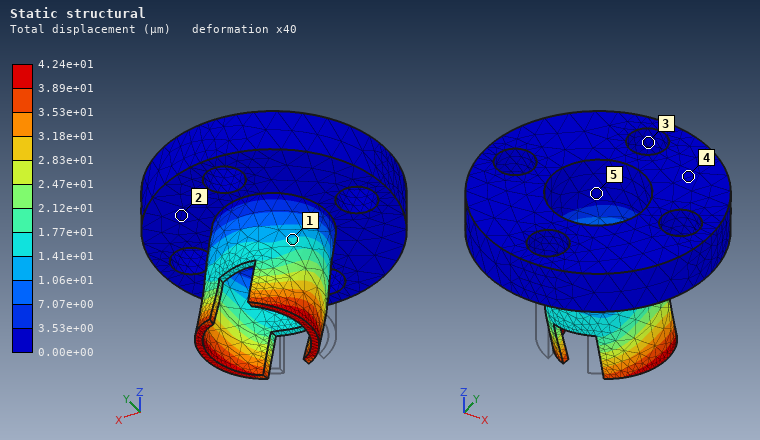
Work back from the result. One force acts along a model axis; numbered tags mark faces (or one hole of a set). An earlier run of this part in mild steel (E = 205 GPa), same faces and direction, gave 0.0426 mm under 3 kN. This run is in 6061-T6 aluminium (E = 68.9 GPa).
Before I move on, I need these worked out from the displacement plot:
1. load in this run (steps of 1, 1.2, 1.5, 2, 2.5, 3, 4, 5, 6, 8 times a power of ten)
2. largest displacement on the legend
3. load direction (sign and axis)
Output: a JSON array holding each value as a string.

["1 kN", "4.24e+01 µm", "+X"]
